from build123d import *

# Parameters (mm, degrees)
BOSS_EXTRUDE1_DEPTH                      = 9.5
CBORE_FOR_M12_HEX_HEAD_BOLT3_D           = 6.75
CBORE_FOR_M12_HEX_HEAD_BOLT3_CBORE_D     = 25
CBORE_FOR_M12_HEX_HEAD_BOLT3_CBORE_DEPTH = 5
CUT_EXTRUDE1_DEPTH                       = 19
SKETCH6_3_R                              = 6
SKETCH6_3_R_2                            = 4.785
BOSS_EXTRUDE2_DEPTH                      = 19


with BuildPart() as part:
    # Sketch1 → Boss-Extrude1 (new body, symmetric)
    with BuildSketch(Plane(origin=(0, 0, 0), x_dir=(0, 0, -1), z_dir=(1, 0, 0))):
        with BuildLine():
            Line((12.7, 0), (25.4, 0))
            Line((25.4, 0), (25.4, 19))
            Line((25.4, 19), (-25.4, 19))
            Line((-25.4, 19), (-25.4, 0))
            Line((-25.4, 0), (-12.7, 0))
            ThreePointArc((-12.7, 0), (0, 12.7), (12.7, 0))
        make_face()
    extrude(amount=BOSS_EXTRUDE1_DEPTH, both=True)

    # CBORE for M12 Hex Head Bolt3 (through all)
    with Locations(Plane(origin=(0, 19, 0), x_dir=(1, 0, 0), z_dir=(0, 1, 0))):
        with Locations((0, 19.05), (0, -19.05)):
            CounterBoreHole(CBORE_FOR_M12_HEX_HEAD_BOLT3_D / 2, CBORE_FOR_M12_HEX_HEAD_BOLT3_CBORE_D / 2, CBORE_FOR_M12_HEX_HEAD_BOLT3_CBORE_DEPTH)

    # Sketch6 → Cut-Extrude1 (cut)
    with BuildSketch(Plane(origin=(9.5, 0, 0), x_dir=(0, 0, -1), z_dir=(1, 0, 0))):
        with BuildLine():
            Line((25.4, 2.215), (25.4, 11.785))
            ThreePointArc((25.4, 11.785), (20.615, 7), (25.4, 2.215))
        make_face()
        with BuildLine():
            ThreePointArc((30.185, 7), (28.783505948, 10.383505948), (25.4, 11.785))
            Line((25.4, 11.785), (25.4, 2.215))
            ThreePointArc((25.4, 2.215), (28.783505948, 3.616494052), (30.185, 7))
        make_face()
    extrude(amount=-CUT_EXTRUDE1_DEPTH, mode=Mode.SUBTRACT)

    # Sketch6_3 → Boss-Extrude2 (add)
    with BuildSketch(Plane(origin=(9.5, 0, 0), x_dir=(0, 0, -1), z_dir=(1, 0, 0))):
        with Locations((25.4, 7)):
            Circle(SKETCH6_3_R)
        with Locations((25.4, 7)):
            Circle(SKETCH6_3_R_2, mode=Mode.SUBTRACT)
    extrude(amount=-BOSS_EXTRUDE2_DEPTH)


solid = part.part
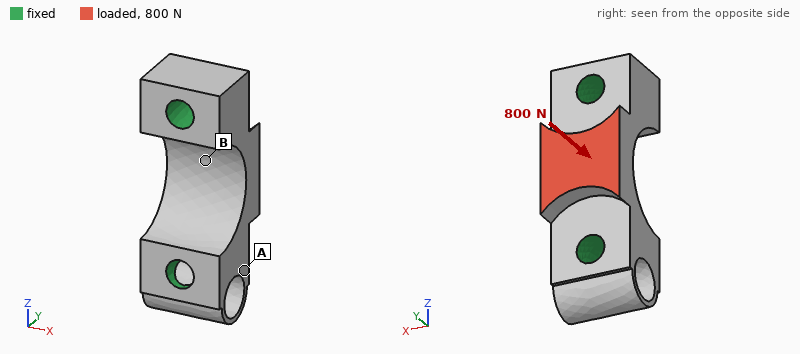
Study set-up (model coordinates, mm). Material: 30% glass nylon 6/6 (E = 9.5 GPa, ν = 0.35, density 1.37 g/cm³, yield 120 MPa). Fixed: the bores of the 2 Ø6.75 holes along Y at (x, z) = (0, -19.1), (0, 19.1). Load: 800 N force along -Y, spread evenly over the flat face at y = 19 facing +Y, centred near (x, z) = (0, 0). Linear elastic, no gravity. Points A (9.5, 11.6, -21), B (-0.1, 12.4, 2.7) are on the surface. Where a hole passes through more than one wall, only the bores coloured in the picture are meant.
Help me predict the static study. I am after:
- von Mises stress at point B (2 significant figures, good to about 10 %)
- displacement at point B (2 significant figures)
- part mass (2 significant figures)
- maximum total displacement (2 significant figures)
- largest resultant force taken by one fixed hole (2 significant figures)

1.7 MPa
19 µm
12 g
21 µm
510 N
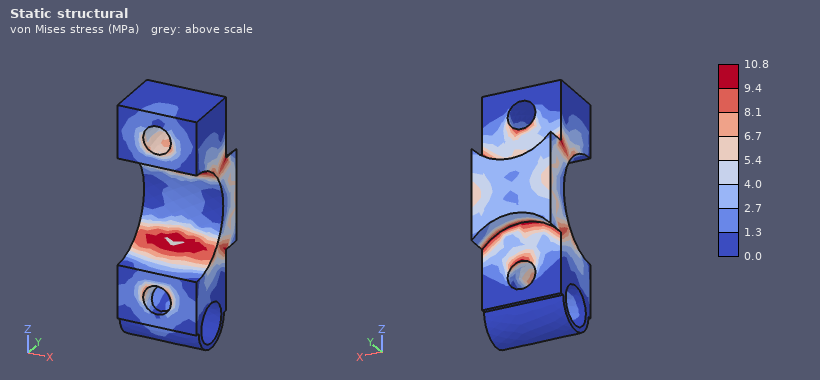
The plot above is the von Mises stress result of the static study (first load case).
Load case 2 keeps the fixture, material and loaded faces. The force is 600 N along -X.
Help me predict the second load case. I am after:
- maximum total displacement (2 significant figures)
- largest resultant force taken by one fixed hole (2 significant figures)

57 µm
310 N
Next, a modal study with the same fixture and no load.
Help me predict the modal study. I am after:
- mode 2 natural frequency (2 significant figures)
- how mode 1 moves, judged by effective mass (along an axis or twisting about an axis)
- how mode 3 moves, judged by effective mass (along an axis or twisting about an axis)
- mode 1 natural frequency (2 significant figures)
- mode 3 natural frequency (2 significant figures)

15 kHz
along X
along Y
12 kHz
18 kHz
